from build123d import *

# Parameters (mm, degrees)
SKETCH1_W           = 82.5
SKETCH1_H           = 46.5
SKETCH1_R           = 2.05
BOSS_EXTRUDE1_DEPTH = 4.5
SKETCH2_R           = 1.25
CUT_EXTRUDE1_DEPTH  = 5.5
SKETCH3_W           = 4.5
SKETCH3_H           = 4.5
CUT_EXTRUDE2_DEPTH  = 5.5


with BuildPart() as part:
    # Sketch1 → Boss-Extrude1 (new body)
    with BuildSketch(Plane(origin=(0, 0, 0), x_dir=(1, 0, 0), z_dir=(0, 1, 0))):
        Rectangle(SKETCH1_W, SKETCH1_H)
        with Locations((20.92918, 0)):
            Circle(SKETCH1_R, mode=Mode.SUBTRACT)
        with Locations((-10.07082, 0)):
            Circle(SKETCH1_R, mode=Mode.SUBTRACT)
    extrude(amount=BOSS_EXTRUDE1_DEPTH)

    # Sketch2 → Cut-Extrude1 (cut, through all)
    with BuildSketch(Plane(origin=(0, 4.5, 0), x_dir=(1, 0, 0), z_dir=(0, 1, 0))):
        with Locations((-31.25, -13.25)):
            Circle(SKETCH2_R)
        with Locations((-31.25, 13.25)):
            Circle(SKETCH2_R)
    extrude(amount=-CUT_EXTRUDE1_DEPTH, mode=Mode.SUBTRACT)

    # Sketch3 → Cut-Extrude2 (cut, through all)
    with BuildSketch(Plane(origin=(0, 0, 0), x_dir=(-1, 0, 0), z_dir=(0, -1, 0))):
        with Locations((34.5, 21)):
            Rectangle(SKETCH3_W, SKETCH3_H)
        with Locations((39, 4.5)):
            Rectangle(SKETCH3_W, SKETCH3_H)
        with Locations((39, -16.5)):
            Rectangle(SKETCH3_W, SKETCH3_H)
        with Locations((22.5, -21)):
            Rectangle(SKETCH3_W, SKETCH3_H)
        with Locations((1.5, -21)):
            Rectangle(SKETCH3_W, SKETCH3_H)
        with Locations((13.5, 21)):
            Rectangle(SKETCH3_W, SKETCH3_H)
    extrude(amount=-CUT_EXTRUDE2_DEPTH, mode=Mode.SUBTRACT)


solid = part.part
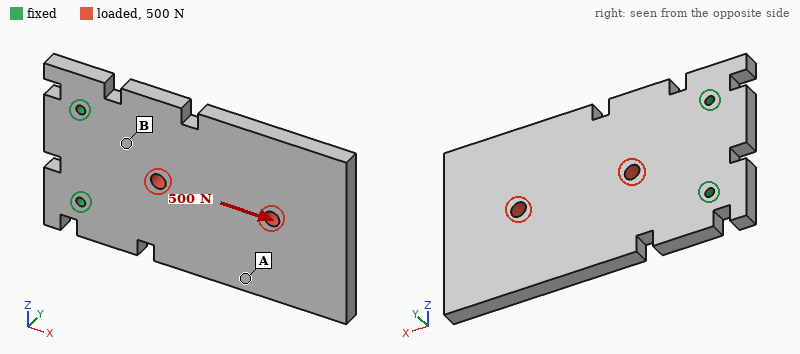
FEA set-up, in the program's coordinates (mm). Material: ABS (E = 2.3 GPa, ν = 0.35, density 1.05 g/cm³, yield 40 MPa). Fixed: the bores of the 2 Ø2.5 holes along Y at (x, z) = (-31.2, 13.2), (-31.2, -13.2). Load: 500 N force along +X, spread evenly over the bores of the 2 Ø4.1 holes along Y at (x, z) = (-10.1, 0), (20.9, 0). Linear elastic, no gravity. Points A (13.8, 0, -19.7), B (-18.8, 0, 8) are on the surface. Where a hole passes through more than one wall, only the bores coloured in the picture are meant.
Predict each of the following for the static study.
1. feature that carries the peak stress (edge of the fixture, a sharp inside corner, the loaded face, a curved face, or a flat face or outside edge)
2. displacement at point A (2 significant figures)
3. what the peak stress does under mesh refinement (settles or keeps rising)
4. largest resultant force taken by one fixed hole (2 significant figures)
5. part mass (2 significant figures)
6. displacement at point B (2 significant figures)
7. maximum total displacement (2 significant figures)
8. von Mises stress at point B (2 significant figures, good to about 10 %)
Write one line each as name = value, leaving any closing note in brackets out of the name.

feature that carries the peak stress = edge of the fixture
displacement at point A = 44 µm
what the peak stress does under mesh refinement = keeps rising
largest resultant force taken by one fixed hole = 250 N
part mass = 17 g
displacement at point B = 27 µm
maximum total displacement = 69 µm
von Mises stress at point B = 3.2 MPa
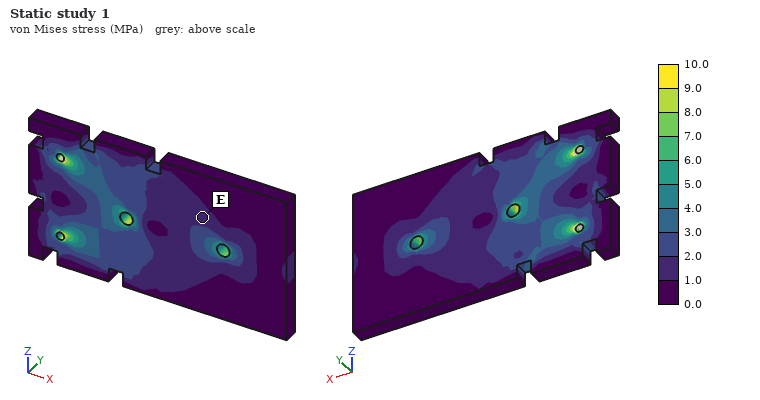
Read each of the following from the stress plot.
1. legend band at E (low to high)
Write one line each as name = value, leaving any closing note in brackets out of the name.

legend band at E = 1.0 to 2.0 MPa
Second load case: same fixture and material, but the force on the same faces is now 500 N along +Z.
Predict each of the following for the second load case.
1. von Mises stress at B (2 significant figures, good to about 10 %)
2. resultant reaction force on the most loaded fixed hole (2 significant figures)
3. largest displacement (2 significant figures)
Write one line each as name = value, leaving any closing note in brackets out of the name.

von Mises stress at B = 8.4 MPa
resultant reaction force on the most loaded fixed hole = 710 N
largest displacement = 0.70 mm
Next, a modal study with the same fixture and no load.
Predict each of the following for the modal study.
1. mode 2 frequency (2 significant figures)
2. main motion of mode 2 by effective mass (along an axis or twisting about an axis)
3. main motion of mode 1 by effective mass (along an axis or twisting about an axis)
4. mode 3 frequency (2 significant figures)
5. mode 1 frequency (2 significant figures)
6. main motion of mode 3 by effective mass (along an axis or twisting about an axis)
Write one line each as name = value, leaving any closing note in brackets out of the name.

mode 2 frequency = 640 Hz
main motion of mode 2 by effective mass = twisting about X
main motion of mode 1 by effective mass = along Y
mode 3 frequency = 1200 Hz
mode 1 frequency = 180 Hz
main motion of mode 3 by effective mass = along Y
